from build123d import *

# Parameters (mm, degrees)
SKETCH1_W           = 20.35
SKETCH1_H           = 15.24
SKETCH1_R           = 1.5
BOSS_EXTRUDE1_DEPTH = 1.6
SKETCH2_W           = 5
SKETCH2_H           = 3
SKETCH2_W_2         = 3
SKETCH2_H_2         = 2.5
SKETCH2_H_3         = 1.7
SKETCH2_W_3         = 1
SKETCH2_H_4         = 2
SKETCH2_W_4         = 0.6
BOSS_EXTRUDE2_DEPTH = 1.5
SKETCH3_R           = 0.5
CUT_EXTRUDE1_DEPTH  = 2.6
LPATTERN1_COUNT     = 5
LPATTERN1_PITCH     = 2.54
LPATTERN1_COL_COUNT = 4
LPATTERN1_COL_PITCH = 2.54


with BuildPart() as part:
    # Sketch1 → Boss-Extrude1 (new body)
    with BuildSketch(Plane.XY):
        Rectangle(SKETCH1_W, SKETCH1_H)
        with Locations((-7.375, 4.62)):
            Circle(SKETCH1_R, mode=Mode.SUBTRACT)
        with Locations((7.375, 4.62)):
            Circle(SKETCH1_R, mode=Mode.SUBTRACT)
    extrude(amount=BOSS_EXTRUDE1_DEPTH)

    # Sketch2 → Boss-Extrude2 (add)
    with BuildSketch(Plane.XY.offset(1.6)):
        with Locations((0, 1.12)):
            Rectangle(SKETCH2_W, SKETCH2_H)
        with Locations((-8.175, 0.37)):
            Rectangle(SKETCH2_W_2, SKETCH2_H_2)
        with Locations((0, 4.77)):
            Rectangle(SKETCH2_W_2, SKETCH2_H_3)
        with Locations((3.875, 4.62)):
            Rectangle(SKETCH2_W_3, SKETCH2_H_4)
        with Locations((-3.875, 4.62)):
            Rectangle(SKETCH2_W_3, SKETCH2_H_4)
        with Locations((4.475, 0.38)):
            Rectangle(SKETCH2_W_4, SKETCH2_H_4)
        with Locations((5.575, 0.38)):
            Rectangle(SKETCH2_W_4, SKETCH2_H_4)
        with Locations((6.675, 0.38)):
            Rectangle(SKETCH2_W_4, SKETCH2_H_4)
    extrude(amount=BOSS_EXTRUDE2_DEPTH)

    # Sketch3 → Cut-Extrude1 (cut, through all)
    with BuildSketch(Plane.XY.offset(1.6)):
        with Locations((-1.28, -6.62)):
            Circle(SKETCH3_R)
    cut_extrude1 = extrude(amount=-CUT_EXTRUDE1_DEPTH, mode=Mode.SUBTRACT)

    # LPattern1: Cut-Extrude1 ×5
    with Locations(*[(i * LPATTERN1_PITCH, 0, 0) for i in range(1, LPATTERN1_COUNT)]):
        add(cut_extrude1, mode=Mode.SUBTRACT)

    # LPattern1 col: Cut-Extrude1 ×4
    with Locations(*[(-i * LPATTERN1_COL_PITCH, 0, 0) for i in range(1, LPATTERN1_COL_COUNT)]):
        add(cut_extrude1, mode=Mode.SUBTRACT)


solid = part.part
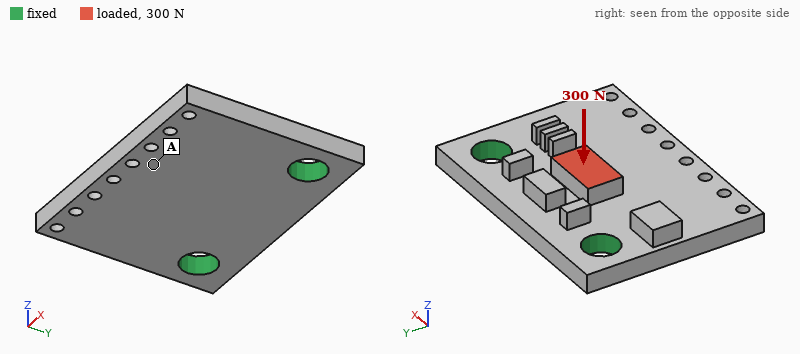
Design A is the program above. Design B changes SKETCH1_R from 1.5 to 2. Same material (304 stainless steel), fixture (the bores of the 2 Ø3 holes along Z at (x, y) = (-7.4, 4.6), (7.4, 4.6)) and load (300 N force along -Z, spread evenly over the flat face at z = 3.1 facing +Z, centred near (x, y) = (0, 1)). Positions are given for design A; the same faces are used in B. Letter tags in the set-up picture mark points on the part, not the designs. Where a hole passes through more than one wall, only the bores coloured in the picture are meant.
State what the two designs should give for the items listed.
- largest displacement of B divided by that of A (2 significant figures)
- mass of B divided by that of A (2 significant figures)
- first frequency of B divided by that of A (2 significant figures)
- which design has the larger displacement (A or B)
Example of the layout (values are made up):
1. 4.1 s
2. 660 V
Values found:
1. 0.73
2. 0.97
3. 1.1
4. A
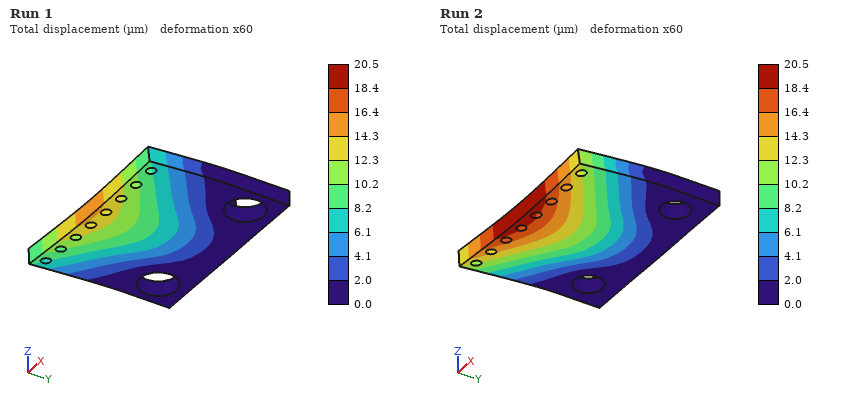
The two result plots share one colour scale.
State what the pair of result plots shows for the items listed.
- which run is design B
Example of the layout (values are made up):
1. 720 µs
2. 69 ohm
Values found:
1. Run 1
